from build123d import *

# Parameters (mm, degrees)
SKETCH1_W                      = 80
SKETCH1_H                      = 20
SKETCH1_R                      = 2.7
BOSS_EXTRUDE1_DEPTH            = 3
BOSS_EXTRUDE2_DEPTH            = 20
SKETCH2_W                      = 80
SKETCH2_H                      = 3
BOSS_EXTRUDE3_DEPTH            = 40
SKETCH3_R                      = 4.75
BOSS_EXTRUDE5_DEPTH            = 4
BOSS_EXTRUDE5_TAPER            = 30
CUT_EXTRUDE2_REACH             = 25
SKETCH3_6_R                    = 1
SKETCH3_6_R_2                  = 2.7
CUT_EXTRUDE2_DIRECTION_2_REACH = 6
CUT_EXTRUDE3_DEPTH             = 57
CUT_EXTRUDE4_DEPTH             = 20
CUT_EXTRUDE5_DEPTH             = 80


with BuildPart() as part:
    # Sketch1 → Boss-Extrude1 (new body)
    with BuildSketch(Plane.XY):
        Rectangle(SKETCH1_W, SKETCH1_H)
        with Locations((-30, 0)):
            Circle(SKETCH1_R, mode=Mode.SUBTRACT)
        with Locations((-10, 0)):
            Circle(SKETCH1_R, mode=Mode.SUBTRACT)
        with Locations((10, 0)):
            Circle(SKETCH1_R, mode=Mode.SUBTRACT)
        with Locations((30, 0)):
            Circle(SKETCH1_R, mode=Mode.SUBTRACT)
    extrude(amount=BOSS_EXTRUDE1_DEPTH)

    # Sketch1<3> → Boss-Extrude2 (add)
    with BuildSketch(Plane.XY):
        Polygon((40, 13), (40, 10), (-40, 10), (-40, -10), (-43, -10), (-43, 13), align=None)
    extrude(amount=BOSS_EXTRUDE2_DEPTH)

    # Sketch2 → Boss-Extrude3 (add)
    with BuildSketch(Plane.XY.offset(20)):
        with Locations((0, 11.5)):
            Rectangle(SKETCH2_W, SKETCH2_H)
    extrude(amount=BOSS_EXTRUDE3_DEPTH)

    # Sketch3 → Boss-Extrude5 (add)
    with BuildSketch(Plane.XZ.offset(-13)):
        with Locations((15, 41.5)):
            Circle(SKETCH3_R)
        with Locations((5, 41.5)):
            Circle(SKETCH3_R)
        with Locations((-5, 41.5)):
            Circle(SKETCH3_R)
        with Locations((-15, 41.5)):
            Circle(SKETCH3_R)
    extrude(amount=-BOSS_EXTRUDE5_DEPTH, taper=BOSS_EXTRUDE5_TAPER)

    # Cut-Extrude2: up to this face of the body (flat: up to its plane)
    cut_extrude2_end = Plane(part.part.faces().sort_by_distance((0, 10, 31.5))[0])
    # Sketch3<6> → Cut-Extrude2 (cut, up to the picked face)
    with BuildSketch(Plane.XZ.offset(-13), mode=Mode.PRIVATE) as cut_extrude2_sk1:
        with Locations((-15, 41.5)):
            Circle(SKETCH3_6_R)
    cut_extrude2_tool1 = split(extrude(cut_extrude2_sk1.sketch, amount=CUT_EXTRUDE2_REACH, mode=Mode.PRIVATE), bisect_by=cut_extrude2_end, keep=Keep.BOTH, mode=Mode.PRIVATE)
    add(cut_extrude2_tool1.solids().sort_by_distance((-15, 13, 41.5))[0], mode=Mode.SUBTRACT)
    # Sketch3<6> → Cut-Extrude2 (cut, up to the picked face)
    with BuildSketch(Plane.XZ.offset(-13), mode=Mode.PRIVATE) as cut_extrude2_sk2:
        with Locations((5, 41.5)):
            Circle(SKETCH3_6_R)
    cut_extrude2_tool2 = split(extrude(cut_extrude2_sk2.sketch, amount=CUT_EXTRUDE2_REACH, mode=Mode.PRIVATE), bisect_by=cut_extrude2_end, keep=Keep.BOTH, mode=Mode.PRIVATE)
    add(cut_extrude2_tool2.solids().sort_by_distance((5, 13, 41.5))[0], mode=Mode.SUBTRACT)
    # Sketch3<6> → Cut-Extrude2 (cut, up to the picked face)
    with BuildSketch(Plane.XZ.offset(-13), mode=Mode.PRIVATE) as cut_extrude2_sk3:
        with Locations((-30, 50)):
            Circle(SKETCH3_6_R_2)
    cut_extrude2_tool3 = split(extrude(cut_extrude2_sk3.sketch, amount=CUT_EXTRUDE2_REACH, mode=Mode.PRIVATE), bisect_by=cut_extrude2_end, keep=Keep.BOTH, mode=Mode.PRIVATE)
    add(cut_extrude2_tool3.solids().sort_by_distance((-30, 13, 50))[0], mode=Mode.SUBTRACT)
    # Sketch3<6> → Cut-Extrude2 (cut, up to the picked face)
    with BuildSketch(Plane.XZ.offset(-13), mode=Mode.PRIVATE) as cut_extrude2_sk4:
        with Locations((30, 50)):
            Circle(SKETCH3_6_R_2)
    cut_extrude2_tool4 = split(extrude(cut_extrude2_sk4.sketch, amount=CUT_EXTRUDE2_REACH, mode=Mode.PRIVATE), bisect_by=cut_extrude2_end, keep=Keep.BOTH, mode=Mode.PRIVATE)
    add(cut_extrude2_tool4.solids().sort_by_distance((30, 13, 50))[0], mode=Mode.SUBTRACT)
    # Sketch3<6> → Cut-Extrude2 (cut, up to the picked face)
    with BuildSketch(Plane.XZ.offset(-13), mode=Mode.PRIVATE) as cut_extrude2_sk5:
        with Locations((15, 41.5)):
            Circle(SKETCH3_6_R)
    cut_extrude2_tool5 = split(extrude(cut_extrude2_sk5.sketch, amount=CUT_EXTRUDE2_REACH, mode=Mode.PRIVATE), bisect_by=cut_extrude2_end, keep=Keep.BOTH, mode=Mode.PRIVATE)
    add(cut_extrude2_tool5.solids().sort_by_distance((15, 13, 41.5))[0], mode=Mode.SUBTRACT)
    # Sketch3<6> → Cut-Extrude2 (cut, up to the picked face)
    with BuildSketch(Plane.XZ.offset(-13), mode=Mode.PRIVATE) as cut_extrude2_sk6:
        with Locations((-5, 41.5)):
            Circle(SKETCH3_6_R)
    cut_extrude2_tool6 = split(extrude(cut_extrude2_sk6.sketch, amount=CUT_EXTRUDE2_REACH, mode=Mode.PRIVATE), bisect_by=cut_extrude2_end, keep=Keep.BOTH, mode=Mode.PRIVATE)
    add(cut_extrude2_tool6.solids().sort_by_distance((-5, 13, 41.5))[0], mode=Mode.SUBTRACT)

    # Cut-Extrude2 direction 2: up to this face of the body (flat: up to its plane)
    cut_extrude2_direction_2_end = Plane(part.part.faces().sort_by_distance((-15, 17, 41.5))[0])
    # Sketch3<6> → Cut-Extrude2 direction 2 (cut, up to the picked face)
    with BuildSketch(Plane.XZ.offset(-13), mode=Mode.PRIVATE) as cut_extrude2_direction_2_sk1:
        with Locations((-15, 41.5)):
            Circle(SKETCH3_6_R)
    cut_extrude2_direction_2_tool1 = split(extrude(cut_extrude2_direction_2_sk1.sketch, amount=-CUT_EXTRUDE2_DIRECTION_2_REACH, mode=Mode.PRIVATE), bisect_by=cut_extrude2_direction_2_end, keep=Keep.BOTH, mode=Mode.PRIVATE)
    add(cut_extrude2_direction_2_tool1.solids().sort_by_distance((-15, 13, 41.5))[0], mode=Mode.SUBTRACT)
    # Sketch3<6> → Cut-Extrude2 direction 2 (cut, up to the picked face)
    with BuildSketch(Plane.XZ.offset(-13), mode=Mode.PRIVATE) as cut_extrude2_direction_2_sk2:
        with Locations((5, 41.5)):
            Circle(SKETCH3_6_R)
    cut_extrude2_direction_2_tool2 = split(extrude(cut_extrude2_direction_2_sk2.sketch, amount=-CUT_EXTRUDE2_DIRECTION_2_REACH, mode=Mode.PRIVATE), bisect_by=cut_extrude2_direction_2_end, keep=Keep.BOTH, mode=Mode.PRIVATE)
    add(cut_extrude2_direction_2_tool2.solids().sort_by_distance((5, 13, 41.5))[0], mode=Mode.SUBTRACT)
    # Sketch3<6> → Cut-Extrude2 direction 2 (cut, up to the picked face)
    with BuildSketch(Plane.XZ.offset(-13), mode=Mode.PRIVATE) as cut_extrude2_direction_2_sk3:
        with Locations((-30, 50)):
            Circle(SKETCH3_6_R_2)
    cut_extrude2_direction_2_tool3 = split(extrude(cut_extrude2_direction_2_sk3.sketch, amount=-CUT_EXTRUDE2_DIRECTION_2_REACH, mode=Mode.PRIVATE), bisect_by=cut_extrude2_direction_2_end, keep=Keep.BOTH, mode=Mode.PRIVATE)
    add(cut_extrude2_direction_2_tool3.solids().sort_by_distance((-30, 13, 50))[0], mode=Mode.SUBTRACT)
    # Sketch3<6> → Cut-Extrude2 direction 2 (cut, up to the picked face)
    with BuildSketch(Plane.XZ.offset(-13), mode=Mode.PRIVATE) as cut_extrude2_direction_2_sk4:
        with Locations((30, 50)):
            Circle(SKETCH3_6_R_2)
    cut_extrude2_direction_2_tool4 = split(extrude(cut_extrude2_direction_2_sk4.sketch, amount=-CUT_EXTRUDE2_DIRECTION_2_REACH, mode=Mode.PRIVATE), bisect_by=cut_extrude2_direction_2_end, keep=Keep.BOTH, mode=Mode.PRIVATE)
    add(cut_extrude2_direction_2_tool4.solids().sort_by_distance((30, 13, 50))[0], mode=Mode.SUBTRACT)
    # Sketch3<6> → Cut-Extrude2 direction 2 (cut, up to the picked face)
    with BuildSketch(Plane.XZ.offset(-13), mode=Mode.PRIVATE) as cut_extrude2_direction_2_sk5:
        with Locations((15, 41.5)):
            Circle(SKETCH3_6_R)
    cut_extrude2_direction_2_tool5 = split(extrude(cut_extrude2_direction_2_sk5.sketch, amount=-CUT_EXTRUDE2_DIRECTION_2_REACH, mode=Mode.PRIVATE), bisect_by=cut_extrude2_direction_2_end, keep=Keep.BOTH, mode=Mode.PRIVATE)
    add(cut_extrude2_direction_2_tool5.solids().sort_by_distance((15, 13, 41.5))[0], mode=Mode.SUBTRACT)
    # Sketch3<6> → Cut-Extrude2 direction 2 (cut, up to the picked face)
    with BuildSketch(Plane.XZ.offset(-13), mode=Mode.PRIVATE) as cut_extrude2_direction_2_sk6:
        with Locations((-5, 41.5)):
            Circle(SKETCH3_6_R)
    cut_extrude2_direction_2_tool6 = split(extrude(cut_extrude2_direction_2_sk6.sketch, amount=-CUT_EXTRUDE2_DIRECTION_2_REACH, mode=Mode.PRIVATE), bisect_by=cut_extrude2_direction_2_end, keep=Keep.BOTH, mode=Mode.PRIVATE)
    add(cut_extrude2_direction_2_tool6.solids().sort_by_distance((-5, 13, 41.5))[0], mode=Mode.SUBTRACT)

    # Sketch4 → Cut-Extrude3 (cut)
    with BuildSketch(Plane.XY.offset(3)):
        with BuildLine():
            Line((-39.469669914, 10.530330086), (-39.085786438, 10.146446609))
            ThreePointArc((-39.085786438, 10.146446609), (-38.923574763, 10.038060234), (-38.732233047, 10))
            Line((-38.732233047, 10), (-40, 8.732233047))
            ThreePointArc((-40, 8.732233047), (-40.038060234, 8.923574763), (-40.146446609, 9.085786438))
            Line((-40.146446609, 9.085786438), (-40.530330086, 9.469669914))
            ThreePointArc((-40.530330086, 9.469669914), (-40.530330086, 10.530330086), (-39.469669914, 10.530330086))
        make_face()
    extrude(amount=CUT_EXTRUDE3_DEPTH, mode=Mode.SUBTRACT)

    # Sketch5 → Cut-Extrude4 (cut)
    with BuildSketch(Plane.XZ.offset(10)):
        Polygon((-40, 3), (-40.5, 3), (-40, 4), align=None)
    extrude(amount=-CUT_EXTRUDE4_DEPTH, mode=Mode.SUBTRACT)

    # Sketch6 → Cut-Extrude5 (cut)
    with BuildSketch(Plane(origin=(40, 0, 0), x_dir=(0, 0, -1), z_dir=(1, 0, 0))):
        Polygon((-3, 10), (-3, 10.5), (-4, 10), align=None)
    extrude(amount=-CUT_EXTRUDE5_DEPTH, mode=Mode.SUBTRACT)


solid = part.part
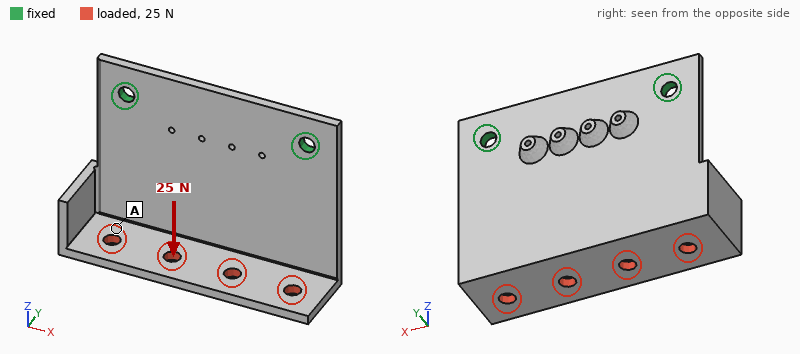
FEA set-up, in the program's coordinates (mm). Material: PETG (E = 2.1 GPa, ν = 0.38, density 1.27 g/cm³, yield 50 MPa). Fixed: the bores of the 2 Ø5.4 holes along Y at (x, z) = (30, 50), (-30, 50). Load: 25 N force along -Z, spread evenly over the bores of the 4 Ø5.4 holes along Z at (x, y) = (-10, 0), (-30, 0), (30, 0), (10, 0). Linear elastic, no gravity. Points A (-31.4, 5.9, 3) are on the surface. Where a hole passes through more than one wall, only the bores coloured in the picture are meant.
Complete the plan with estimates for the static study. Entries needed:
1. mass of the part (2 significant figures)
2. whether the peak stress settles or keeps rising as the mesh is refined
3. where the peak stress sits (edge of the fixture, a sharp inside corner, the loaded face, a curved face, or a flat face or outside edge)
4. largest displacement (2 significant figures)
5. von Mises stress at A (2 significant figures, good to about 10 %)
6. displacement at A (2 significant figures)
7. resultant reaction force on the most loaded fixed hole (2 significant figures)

26 g
keeps rising
a sharp inside corner
1.2 mm
0.68 MPa
0.89 mm
13 N
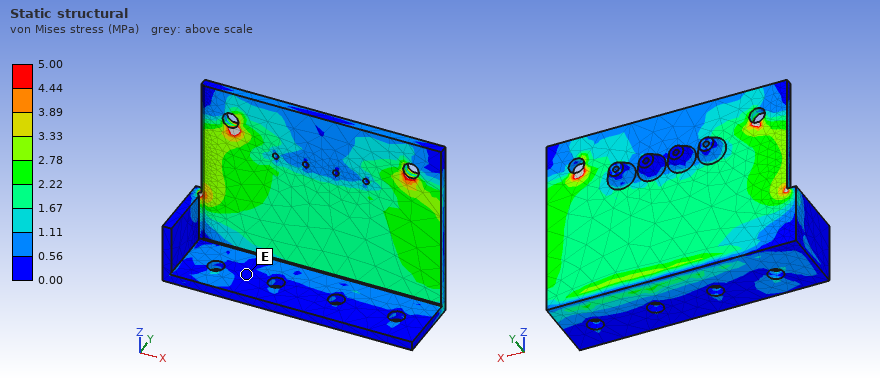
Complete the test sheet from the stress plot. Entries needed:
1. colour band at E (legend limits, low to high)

0.00 to 0.56 MPa
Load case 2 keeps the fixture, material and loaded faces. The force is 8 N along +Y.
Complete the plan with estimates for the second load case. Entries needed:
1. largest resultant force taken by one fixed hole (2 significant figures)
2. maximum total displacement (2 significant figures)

4.4 N
1.0 mm
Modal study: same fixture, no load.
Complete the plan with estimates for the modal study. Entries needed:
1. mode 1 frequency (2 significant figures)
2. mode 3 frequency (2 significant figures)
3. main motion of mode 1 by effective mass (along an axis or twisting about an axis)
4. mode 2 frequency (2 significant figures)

140 Hz
680 Hz
along Y
270 Hz
